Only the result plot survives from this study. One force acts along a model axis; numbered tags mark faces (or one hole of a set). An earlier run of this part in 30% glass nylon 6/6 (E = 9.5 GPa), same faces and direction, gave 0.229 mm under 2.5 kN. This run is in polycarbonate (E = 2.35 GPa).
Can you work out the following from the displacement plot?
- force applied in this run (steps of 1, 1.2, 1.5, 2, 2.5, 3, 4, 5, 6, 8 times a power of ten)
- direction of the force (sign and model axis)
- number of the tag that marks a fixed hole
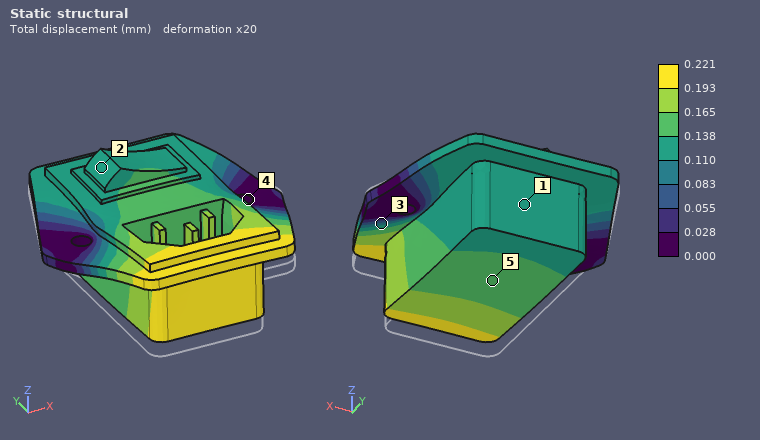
600 N
+Z
4
